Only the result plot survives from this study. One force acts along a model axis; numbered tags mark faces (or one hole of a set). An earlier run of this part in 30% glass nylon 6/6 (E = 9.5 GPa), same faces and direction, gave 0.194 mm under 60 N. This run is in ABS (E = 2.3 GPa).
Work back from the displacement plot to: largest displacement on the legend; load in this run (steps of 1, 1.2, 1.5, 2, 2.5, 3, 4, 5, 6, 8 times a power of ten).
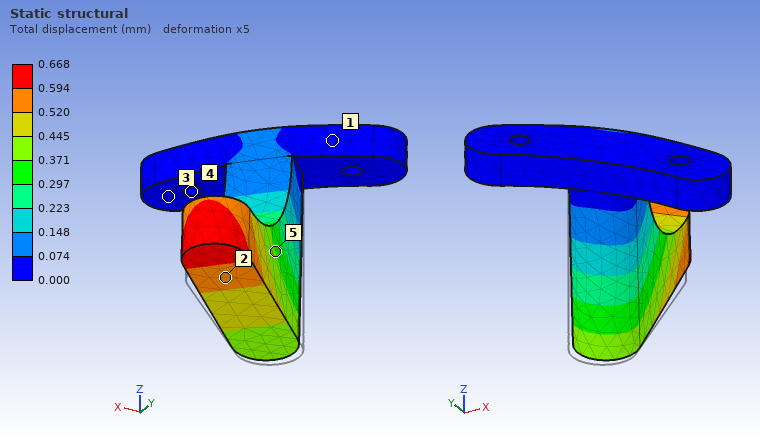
0.668 mm
50 N
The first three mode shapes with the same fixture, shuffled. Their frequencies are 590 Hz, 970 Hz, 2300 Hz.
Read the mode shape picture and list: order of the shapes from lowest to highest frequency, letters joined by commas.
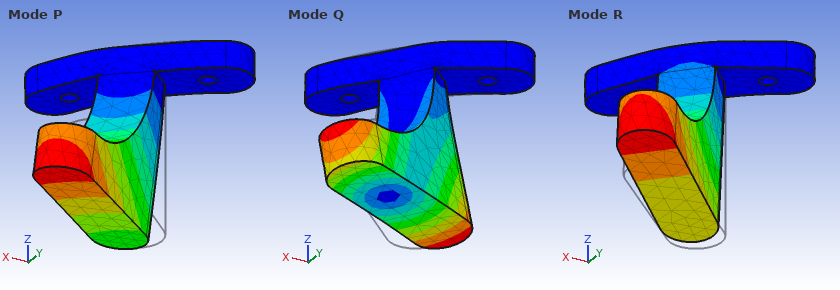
R, P, Q
